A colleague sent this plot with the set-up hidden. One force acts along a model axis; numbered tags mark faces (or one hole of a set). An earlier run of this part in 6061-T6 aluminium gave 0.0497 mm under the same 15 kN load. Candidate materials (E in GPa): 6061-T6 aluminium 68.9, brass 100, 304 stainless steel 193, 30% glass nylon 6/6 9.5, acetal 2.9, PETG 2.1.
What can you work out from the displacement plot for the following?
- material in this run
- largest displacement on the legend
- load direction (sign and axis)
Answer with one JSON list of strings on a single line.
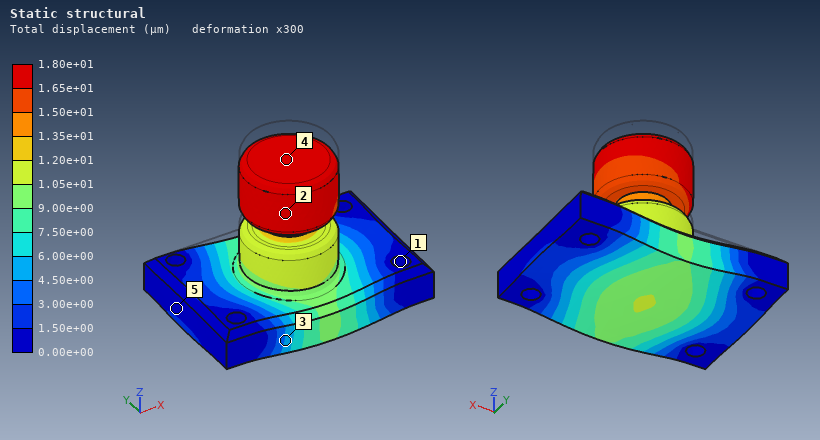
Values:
["304 stainless steel", "1.80e+01 µm", "-Z"]
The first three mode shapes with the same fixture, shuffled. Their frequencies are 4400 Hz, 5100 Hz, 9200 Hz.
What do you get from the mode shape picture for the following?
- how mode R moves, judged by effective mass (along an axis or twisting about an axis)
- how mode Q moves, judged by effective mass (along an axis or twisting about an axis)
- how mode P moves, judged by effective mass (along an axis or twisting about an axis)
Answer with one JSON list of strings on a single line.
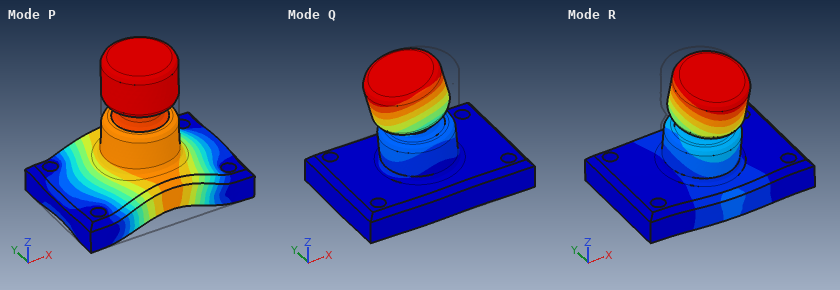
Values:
["along Y", "along X", "along Z"]
